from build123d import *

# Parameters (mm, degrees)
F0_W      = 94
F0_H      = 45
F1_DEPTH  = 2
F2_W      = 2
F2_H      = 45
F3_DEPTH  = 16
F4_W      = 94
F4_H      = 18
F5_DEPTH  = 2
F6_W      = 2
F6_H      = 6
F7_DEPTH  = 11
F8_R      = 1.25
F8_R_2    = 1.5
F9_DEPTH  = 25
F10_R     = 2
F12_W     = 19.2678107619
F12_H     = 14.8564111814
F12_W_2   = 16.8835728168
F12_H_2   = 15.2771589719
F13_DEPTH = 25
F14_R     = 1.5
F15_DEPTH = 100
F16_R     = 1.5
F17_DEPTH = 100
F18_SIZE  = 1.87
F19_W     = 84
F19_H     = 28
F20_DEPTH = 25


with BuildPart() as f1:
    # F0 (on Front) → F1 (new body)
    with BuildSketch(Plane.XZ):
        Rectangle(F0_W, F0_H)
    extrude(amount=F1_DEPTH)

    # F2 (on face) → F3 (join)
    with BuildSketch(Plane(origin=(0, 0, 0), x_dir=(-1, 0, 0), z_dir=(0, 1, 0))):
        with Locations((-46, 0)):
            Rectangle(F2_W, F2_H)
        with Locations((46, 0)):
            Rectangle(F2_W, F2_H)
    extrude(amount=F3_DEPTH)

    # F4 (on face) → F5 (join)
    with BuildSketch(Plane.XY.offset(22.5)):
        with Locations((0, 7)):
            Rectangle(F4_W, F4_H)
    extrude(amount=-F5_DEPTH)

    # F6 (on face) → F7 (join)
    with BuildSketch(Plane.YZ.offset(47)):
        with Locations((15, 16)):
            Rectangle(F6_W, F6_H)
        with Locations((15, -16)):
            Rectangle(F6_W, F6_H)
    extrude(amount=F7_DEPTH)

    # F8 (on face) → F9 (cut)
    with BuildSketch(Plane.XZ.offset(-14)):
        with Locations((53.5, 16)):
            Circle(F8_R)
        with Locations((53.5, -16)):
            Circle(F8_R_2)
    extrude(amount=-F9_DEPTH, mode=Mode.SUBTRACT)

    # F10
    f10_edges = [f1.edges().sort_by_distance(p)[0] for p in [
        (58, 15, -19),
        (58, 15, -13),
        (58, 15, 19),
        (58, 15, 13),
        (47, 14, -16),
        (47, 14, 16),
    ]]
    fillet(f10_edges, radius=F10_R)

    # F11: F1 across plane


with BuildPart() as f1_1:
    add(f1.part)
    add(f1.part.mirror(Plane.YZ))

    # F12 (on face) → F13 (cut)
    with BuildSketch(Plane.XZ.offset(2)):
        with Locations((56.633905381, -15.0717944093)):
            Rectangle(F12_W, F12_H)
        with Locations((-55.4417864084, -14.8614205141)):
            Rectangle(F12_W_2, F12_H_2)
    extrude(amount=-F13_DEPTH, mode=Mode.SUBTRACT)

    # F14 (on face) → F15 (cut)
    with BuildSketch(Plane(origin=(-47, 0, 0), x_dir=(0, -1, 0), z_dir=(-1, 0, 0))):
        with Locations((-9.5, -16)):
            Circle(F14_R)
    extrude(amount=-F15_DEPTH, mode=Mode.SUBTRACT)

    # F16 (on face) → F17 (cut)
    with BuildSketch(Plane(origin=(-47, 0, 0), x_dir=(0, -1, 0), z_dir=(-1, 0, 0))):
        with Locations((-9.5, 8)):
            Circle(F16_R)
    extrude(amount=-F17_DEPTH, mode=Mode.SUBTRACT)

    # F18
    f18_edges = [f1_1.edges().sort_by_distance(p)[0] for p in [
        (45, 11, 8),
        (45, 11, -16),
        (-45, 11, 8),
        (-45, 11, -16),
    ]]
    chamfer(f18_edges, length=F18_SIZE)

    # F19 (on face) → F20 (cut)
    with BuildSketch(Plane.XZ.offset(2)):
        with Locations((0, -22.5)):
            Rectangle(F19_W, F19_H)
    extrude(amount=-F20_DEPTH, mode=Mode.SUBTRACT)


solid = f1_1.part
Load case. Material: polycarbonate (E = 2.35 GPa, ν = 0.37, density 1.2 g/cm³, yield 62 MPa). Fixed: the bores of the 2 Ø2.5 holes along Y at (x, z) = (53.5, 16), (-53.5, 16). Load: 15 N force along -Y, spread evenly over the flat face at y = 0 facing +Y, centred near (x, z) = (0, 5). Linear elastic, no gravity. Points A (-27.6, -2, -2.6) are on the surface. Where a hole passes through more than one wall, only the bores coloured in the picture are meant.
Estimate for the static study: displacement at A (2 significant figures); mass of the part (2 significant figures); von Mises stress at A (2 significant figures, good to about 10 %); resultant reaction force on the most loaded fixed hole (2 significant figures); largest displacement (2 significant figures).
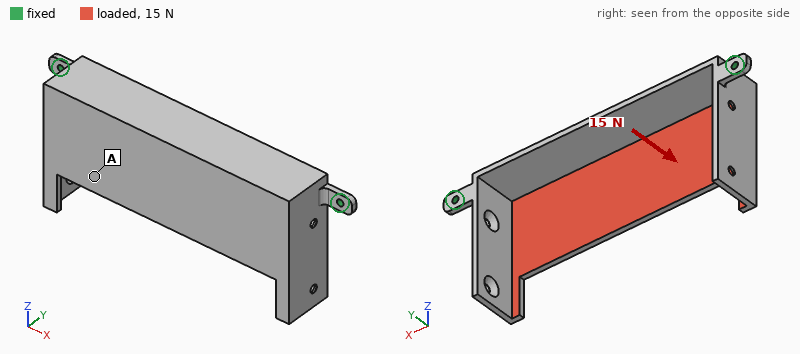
1.0 mm
14 g
1.5 MPa
9.3 N
1.4 mm
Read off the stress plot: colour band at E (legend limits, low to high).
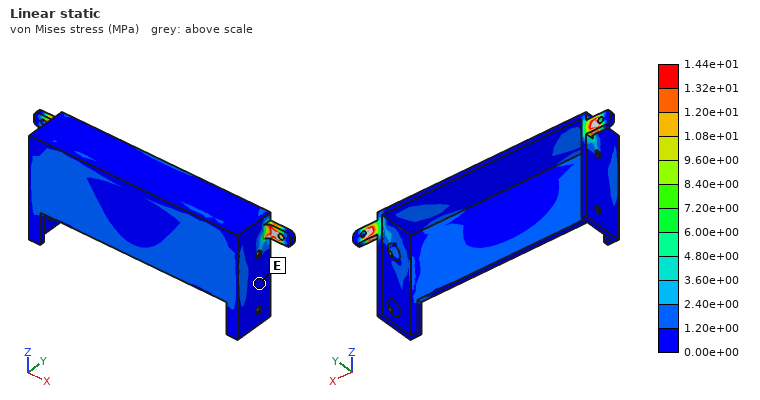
0.00e+00 to 1.20e+00 MPa
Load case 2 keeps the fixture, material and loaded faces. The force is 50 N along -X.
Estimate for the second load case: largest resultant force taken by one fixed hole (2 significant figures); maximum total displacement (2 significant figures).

27 N
1.3 mm
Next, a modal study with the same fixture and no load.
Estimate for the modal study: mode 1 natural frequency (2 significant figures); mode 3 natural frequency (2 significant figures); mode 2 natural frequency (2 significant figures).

150 Hz
470 Hz
270 Hz
